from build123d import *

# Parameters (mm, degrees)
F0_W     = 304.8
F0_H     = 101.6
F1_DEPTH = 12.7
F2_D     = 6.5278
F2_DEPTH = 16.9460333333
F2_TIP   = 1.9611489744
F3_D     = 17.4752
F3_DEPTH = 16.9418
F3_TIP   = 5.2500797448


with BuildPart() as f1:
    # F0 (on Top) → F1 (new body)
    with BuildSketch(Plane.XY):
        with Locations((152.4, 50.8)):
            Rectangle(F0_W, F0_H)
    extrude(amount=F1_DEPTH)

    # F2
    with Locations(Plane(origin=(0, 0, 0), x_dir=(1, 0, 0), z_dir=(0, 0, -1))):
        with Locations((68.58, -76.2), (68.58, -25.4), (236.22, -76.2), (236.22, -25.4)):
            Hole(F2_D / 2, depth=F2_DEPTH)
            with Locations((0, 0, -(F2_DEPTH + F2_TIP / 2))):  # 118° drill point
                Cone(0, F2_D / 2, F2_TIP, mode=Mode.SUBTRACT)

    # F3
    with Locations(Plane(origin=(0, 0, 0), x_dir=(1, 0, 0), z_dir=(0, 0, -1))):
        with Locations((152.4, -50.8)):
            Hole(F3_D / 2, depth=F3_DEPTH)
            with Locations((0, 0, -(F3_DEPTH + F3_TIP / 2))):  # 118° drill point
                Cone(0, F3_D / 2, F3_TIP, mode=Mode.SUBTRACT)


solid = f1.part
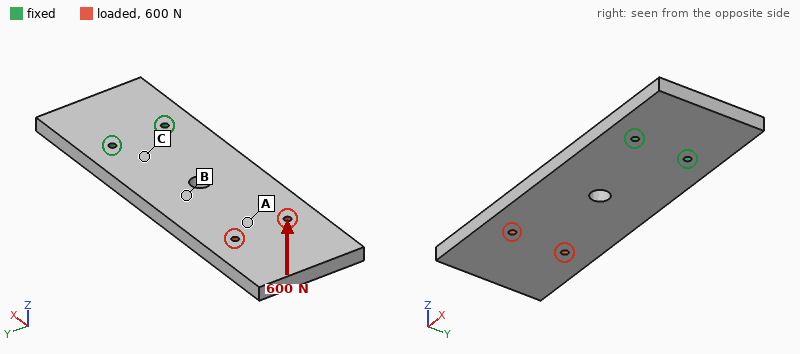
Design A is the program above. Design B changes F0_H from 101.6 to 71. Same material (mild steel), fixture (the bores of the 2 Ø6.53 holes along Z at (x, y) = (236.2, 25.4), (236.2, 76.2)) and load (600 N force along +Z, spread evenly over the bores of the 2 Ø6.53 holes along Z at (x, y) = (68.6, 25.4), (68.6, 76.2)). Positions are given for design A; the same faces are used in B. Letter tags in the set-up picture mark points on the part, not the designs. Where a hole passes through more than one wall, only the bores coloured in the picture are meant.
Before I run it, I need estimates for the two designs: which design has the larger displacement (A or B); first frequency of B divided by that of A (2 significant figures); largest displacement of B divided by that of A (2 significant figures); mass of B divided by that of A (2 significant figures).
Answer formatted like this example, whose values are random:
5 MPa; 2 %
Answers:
B; 1.0; 1.4; 0.70
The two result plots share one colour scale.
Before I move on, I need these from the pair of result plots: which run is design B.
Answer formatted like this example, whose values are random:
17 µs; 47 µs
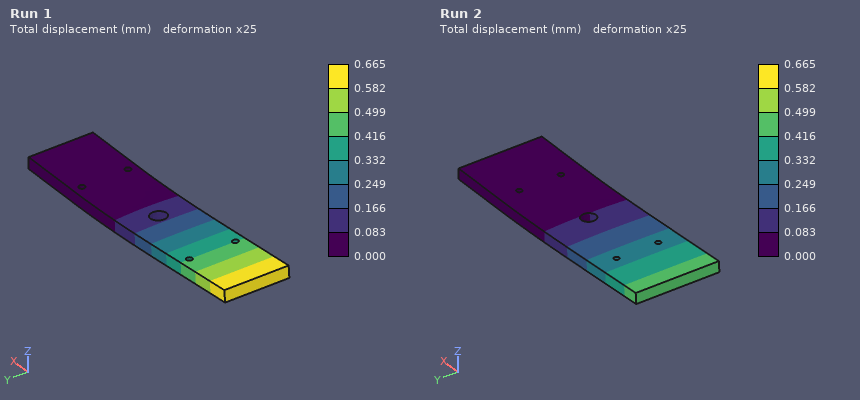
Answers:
Run 1
